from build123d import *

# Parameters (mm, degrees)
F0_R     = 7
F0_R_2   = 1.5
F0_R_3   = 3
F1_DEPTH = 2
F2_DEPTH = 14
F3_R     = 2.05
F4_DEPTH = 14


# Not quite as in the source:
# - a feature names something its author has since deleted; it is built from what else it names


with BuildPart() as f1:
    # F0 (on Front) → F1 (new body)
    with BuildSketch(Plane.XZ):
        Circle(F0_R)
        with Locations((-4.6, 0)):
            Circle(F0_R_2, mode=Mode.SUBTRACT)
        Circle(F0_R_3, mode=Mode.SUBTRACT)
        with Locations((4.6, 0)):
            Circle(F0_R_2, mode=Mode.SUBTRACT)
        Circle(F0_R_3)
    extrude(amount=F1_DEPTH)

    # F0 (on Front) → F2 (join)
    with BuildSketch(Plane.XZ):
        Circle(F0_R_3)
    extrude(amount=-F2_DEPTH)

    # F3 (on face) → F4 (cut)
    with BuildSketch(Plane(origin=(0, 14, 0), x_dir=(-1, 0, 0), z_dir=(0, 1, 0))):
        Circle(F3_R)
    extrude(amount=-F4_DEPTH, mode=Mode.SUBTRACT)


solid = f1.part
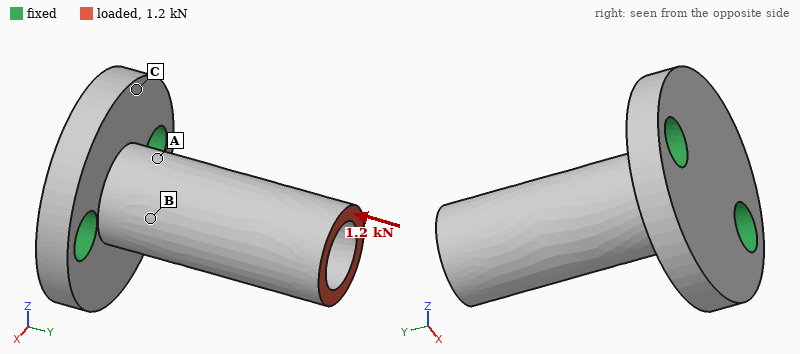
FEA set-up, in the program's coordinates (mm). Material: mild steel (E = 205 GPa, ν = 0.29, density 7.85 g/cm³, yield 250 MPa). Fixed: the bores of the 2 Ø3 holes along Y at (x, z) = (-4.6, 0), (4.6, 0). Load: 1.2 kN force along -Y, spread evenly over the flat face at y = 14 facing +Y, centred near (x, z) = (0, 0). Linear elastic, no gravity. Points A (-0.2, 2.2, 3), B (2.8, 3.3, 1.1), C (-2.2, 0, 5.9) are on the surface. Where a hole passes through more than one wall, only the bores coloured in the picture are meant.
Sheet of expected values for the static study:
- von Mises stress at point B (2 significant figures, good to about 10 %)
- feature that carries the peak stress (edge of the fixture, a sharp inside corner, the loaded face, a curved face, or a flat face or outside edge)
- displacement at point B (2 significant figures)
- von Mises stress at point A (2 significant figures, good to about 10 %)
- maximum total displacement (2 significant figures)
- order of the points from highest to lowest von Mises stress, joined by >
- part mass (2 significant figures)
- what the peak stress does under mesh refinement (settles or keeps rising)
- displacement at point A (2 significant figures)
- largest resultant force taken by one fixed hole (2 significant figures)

86 MPa
edge of the fixture
2.7 µm
52 MPa
6.9 µm
B > A > C
3.9 g
keeps rising
2.6 µm
610 N
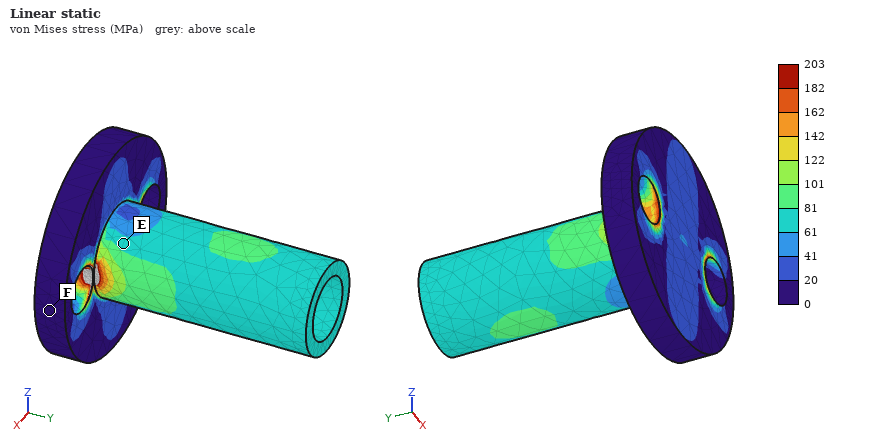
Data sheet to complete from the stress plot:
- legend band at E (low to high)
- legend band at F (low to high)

61 to 81 MPa
0 to 20 MPa
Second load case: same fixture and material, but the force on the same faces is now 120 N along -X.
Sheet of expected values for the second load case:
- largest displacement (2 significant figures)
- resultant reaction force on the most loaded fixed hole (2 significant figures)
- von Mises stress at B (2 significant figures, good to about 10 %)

17 µm
280 N
71 MPa
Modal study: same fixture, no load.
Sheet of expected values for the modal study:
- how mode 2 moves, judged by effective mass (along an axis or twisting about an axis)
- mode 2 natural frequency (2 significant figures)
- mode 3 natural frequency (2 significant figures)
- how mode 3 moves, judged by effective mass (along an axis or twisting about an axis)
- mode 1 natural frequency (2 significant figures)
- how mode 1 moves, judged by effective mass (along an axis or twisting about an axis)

along X
20 kHz
54 kHz
along Y
15 kHz
along Z
